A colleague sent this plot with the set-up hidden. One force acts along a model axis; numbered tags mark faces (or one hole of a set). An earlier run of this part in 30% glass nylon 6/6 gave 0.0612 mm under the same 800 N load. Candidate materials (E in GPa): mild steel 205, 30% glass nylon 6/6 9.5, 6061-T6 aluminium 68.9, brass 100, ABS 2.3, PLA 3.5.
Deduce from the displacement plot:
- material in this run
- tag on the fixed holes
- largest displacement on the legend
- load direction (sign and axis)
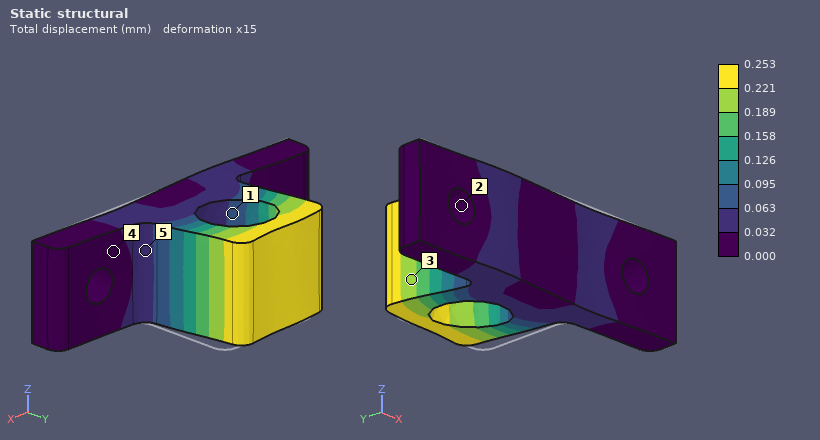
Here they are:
ABS
2
0.253 mm
-X
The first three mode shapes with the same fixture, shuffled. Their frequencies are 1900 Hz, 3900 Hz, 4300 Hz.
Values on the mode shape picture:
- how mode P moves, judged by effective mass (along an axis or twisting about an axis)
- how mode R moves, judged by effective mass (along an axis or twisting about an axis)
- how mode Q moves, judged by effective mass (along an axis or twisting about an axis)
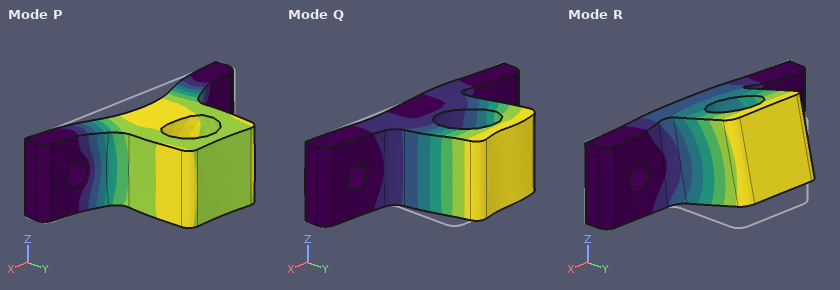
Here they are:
along Y
along Z
along X
